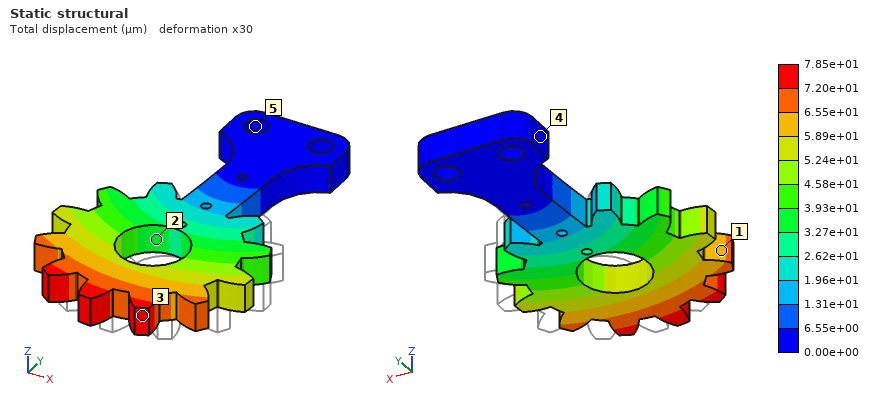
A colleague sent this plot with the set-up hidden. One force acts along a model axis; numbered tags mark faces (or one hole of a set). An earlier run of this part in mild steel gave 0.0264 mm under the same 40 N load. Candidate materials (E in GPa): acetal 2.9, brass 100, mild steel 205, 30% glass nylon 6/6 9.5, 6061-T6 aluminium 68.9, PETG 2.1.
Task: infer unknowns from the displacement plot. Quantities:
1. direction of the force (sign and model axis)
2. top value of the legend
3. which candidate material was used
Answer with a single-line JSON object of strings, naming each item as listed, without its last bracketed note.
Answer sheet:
{"direction of the force": "-X", "top value of the legend": "7.85e+01 µm", "which candidate material was used": "6061-T6 aluminium"}
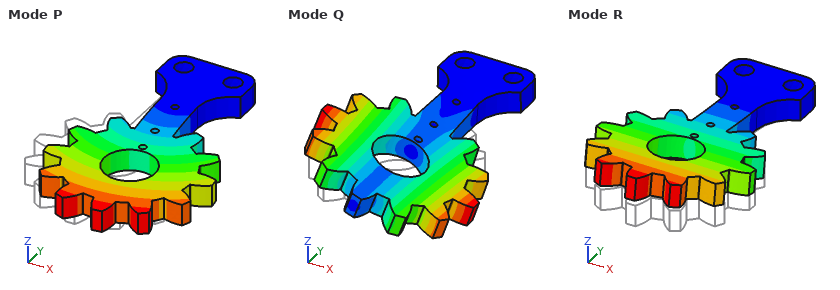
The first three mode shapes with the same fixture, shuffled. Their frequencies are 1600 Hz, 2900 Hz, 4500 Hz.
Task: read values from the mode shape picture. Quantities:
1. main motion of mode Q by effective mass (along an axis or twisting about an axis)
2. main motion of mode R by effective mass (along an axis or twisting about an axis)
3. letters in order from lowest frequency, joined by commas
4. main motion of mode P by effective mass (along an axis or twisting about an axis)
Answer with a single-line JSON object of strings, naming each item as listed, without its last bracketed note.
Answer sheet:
{"main motion of mode Q by effective mass": "twisting about Y", "main motion of mode R by effective mass": "along Z", "letters in order from lowest frequency, joined by commas": "R, P, Q", "main motion of mode P by effective mass": "along X"}
